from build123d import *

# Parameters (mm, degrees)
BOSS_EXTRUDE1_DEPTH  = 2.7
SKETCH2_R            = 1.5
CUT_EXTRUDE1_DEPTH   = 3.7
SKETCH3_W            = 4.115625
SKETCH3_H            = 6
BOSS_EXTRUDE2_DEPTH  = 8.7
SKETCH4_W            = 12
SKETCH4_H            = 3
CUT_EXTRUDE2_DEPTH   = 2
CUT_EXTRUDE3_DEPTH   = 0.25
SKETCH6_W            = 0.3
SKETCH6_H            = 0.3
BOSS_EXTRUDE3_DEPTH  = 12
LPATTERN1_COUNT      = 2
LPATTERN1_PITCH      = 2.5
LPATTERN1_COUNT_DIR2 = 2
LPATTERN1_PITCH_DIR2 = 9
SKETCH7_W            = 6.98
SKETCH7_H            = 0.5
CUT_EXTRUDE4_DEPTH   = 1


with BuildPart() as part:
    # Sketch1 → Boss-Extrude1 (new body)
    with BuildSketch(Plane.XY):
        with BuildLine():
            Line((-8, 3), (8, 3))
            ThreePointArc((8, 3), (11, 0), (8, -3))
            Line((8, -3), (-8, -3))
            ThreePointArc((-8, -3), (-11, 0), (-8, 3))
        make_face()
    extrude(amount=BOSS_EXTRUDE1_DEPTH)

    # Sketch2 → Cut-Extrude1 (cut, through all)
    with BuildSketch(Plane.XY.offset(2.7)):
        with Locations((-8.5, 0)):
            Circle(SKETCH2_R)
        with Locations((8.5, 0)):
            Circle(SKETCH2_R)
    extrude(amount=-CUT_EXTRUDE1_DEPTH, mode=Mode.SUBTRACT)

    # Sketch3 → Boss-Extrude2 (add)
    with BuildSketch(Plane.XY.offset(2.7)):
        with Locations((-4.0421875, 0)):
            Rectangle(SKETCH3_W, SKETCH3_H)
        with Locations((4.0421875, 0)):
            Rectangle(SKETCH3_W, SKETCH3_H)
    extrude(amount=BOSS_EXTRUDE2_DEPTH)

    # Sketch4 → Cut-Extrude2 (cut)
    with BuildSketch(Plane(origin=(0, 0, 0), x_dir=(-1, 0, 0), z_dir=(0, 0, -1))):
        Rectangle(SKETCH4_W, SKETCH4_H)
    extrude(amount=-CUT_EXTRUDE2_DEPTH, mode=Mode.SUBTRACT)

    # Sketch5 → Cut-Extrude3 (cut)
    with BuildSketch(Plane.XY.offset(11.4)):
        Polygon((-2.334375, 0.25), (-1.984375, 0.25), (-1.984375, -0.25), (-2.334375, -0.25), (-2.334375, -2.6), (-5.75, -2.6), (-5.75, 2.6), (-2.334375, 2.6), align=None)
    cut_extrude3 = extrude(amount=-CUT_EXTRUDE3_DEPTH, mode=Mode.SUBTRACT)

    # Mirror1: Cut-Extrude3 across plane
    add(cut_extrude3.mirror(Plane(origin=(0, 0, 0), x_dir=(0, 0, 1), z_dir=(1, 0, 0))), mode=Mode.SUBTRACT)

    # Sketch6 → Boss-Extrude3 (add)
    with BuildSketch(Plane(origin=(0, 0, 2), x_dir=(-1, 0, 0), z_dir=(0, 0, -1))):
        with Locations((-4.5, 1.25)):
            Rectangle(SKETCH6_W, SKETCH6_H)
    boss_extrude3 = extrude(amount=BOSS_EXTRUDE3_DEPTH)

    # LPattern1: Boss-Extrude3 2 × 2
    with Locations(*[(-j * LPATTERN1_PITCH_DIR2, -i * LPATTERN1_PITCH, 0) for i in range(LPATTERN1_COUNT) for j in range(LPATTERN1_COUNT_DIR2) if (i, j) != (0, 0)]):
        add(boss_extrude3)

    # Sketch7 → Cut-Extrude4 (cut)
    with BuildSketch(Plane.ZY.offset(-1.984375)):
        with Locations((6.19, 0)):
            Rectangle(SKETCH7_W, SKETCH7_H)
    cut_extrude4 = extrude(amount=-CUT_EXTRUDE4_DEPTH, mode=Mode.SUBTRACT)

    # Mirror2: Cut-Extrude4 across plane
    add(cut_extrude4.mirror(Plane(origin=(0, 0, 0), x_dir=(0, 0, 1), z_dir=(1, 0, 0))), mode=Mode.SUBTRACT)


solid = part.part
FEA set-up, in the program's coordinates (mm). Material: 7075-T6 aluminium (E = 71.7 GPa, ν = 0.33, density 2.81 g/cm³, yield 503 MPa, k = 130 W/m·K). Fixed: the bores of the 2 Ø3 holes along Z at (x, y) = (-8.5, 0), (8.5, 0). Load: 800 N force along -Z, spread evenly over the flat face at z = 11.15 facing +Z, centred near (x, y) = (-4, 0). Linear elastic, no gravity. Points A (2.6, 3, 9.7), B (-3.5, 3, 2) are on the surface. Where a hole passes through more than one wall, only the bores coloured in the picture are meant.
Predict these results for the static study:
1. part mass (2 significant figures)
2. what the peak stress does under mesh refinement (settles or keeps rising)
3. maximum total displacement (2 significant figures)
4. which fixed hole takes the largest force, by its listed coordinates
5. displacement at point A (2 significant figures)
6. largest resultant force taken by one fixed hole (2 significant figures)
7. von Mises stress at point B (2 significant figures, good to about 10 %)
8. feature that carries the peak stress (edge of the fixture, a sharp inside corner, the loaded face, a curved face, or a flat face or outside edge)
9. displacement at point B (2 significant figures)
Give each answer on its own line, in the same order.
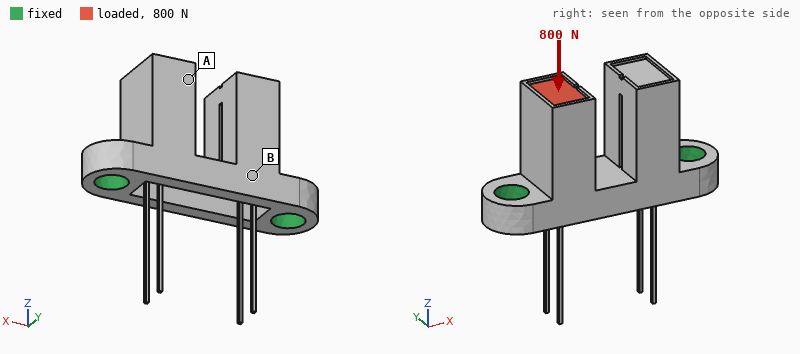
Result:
1.8 g
keeps rising
57 µm
(-8.5, 0)
28 µm
660 N
52 MPa
edge of the fixture
18 µm
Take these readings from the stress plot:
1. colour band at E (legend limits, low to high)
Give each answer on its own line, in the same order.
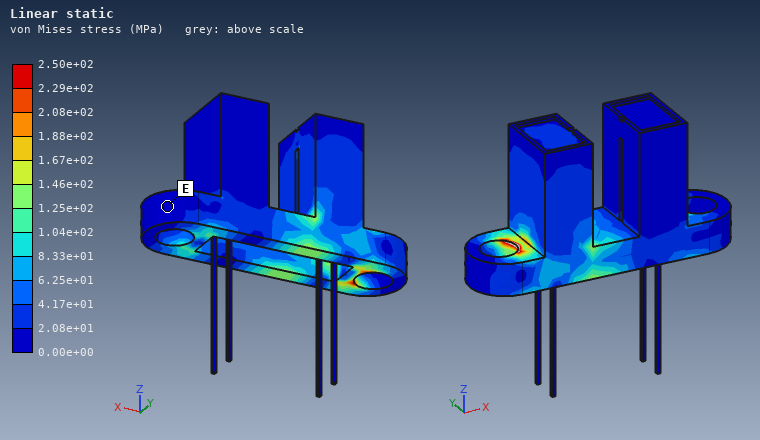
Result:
0.00e+00 to 2.08e+01 MPa
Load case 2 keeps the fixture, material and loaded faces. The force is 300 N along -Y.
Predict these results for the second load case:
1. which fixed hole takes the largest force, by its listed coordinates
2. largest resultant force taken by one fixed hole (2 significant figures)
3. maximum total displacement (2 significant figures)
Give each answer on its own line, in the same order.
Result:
(-8.5, 0)
240 N
87 µm
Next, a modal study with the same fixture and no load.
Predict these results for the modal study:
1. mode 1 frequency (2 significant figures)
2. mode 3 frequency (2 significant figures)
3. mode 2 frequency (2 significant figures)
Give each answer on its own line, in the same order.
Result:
1700 Hz
1700 Hz
1700 Hz
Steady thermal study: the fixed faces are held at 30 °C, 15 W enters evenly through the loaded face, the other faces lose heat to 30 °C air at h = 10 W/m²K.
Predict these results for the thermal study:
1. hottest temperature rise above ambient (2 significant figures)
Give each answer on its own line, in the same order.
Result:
63 K
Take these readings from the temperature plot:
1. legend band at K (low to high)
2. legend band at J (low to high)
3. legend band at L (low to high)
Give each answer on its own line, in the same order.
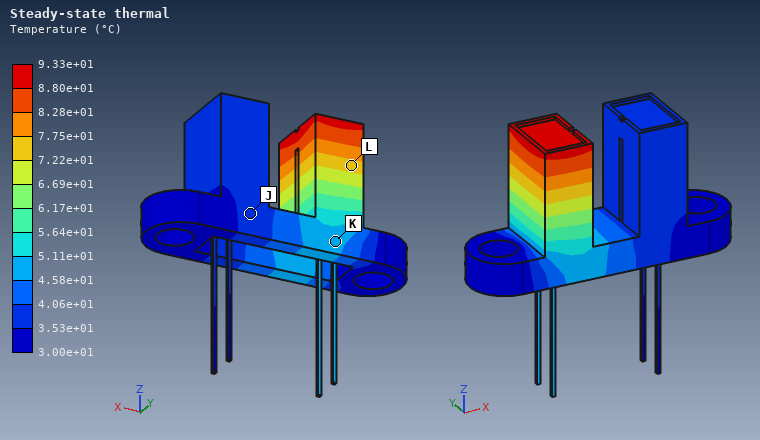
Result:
4.58e+01 to 5.11e+01 °C
3.53e+01 to 4.06e+01 °C
7.22e+01 to 7.75e+01 °C
